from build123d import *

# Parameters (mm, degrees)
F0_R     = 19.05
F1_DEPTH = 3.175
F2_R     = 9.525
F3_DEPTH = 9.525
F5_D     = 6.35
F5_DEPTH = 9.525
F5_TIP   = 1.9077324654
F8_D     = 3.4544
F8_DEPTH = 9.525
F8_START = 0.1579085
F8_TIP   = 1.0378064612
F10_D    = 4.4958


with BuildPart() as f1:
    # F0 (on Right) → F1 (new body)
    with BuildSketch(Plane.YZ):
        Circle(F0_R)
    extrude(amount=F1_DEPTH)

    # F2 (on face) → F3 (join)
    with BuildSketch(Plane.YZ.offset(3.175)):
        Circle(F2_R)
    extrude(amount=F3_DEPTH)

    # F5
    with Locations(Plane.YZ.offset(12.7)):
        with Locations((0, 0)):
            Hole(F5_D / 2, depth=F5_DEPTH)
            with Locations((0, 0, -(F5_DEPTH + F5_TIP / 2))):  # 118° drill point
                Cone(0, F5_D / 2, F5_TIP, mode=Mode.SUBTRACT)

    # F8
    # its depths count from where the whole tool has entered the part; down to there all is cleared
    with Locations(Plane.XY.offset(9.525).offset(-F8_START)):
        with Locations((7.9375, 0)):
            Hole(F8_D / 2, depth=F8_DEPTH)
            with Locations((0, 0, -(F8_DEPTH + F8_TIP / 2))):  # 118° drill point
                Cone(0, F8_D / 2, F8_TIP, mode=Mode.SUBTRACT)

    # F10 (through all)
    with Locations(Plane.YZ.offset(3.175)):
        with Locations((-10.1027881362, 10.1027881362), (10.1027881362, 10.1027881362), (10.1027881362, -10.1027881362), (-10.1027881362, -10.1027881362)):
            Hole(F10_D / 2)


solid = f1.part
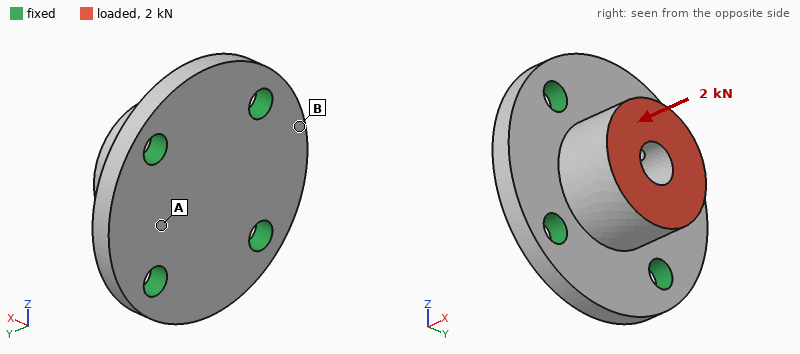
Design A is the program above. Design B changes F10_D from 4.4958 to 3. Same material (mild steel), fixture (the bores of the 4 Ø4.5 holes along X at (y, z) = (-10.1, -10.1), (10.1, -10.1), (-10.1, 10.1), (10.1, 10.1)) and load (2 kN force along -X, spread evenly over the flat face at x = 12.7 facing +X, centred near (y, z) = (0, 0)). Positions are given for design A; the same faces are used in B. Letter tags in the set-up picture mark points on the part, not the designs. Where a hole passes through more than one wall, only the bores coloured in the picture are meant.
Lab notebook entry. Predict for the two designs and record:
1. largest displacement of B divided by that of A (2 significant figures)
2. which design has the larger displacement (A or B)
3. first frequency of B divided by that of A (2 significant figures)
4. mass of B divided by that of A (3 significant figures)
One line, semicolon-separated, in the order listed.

1.3; B; 0.86; 1.02
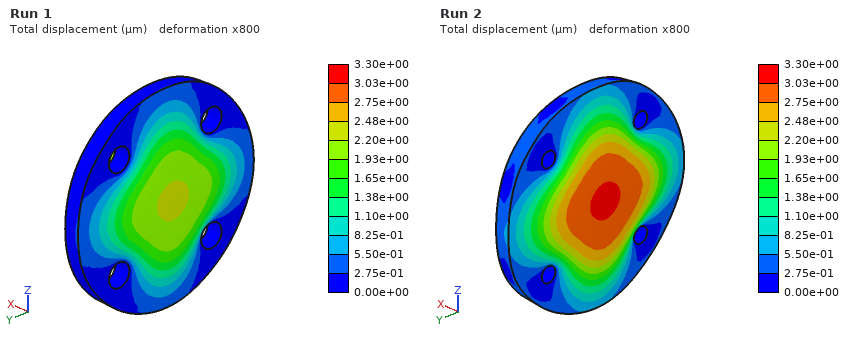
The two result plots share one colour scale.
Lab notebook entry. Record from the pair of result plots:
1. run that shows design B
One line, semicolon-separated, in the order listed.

Run 2
